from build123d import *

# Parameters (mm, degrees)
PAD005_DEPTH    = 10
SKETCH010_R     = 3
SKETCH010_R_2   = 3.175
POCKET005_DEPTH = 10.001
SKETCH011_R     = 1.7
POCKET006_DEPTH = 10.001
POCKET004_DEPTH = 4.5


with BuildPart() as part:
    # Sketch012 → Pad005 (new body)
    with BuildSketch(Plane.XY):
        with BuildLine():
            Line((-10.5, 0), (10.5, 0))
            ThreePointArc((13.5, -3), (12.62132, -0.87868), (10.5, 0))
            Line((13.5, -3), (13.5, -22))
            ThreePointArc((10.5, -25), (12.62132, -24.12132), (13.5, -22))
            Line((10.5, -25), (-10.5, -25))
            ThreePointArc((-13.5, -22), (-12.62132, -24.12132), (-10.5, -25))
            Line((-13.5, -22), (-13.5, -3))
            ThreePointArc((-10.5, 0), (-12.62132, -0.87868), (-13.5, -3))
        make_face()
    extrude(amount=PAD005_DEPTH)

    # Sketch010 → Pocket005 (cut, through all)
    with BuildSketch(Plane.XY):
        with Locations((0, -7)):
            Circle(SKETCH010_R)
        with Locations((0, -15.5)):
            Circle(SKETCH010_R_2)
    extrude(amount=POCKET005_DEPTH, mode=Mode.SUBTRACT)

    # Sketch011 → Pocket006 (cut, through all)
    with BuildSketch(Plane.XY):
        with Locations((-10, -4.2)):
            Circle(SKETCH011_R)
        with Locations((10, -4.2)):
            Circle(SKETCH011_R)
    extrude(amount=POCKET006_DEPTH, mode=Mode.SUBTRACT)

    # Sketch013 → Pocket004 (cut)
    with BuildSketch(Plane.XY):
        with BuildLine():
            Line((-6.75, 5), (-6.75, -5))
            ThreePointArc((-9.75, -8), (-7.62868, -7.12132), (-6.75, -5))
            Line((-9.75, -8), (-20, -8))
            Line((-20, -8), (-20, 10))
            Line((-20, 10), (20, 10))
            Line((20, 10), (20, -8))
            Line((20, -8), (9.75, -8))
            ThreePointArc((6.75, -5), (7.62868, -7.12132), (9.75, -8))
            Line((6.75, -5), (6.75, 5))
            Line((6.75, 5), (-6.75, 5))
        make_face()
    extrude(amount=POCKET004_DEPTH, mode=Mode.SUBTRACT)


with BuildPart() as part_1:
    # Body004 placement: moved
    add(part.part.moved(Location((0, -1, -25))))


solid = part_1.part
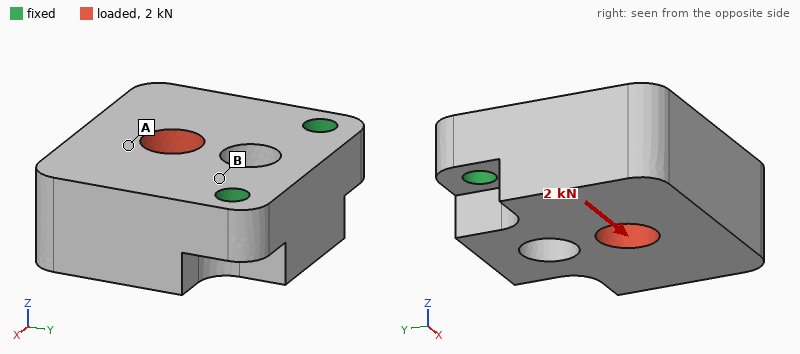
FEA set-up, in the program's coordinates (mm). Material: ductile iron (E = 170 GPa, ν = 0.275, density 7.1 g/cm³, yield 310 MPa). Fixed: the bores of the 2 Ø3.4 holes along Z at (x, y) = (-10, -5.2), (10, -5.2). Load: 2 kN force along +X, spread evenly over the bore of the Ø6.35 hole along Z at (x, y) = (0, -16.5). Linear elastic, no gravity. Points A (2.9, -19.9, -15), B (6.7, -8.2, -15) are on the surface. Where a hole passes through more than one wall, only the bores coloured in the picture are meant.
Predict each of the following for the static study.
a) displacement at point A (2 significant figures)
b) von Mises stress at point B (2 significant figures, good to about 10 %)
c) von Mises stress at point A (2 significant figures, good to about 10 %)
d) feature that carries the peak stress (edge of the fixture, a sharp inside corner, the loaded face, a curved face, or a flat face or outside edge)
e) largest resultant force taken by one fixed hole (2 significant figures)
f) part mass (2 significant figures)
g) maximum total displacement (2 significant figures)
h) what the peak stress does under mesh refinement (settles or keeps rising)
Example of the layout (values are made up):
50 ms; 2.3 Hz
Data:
4.4 µm; 30 MPa; 12 MPa; edge of the fixture; 1.4 kN; 39 g; 5.0 µm; keeps rising
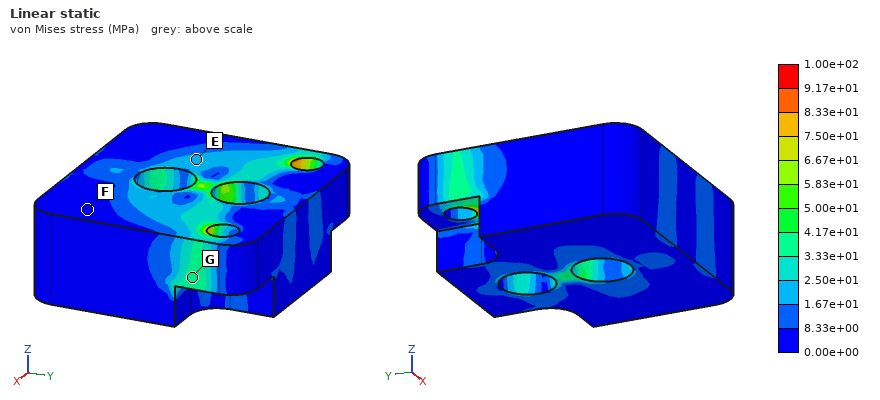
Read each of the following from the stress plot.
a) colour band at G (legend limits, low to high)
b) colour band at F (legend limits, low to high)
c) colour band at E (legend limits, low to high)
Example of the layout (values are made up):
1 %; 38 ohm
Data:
3.33e+01 to 4.17e+01 MPa; 0.00e+00 to 8.33e+00 MPa; 1.67e+01 to 2.50e+01 MPa
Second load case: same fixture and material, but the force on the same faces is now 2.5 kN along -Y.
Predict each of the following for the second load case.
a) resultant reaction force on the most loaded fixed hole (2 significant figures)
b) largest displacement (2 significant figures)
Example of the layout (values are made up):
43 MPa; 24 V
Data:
1.3 kN; 9.3 µm
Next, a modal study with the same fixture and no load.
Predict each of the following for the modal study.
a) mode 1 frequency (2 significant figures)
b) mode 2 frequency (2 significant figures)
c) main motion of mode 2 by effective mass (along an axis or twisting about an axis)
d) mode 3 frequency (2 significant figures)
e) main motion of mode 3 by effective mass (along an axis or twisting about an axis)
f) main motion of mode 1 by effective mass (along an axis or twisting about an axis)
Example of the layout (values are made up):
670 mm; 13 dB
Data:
8000 Hz; 19 kHz; along X; 21 kHz; along X; along Z
